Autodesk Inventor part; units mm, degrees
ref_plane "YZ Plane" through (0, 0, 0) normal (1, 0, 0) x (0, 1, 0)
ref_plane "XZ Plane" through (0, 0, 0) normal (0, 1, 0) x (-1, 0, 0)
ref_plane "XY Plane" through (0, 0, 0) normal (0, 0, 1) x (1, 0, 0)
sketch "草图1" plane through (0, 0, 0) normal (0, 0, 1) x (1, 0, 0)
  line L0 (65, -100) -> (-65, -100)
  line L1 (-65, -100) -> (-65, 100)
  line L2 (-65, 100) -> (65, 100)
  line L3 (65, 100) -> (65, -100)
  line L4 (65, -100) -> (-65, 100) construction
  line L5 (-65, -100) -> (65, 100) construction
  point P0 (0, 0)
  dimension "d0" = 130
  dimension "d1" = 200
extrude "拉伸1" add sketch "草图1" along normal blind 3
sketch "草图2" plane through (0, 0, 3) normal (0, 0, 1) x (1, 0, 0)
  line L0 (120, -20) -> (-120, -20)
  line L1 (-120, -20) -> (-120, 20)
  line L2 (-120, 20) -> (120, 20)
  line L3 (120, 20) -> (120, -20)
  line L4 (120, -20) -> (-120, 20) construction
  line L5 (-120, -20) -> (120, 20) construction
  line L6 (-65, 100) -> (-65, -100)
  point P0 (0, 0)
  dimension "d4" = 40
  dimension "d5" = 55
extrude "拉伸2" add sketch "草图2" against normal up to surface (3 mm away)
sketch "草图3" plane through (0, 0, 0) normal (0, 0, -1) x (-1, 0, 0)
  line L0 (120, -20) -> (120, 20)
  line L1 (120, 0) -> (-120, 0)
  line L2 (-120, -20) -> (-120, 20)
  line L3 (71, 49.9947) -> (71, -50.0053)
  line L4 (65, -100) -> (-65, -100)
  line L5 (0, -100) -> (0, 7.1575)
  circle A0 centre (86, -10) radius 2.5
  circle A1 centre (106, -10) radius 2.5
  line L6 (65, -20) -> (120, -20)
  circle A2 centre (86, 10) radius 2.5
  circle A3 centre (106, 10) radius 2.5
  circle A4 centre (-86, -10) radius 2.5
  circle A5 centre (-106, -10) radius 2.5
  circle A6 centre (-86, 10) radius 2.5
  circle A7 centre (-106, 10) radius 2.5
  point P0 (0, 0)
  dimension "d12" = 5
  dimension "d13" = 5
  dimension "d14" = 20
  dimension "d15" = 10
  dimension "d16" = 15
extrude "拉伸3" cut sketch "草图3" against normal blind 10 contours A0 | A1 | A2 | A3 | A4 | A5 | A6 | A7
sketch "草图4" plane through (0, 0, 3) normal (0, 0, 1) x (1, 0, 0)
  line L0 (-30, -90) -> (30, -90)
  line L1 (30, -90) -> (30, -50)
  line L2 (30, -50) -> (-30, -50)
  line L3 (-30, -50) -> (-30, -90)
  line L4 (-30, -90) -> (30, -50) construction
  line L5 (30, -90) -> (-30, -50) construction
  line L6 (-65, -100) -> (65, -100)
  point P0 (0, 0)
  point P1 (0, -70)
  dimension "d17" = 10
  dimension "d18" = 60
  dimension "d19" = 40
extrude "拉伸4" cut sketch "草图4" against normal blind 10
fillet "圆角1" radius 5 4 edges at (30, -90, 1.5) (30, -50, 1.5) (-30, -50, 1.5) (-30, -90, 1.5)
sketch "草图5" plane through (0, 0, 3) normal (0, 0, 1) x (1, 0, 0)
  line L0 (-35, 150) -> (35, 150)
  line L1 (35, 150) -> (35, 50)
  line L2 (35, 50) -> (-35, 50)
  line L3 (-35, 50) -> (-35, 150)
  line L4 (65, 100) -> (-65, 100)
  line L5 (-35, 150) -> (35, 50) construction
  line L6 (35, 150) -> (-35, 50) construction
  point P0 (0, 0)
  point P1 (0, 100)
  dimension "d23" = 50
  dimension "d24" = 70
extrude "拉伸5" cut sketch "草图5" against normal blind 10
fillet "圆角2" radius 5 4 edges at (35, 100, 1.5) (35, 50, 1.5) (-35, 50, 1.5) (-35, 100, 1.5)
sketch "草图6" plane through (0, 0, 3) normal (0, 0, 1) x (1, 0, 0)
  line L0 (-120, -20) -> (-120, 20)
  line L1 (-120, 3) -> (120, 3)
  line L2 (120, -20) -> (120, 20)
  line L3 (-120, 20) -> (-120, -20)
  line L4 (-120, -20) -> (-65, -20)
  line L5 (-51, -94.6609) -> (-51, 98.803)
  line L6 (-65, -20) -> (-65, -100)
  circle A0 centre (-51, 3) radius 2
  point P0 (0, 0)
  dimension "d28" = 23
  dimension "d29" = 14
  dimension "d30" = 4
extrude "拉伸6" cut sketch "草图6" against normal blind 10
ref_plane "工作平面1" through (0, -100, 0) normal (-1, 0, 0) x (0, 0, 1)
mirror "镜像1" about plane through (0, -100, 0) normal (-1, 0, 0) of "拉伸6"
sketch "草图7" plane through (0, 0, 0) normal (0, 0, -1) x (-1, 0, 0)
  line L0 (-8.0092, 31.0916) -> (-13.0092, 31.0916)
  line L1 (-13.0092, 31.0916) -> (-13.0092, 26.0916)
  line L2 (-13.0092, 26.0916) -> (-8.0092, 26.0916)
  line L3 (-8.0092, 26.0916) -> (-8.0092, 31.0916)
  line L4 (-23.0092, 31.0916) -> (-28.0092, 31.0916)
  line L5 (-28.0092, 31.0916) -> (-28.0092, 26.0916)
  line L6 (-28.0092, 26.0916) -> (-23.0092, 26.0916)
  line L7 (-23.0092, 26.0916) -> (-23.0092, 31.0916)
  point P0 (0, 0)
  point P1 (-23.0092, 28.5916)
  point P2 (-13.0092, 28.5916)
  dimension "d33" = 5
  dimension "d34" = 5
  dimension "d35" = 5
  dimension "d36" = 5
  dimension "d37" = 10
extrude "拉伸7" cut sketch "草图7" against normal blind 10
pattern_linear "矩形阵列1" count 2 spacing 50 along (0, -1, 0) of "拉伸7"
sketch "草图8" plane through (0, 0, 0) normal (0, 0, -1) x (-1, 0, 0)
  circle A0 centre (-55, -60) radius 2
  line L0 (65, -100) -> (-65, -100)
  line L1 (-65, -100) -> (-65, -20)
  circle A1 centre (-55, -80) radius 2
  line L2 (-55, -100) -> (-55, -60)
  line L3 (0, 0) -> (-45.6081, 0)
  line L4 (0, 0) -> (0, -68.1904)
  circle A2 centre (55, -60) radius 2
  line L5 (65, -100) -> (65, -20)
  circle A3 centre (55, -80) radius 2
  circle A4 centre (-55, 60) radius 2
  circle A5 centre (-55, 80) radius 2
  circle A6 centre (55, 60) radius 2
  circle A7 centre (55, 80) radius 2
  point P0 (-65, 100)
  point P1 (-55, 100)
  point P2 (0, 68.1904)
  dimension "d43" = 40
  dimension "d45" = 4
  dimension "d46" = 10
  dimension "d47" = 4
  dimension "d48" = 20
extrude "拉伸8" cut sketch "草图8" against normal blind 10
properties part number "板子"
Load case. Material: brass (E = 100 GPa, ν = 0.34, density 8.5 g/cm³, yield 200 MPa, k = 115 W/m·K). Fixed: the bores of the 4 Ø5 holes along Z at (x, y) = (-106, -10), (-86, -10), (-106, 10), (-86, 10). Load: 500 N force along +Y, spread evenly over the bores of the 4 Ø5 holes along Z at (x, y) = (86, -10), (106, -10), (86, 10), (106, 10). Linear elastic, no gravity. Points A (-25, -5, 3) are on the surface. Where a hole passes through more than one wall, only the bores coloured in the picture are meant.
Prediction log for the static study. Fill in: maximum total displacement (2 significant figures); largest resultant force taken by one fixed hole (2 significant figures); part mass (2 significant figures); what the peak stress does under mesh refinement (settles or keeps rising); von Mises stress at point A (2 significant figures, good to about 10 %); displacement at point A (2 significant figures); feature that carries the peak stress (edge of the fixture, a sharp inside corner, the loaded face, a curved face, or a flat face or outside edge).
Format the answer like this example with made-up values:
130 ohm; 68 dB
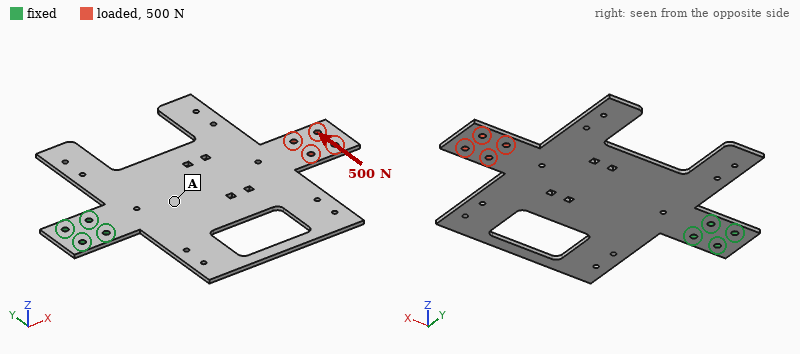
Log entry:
0.45 mm; 3.1 kN; 620 g; keeps rising; 12 MPa; 0.10 mm; edge of the fixture
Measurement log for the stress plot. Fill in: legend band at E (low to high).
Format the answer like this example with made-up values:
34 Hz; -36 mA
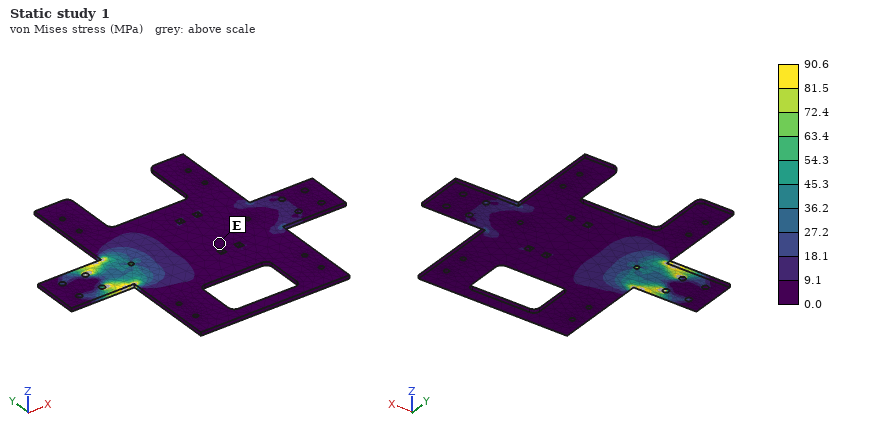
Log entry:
0.0 to 9.1 MPa
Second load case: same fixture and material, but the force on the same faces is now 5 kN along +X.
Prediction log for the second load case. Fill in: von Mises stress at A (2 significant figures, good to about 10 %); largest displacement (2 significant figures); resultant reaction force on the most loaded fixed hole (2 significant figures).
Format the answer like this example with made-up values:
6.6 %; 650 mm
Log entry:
27 MPa; 60 µm; 2.2 kN
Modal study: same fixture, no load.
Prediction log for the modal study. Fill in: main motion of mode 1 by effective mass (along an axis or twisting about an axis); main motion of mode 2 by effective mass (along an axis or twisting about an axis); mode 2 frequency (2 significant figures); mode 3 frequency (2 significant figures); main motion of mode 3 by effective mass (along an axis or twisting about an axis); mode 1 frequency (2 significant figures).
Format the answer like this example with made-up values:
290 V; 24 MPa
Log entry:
along Z; twisting about X; 79 Hz; 190 Hz; along Z; 36 Hz
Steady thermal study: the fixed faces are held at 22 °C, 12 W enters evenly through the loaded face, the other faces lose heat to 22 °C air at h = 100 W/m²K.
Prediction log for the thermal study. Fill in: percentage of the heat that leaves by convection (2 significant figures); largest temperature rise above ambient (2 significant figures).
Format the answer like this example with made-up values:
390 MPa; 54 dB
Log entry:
99 %; 20 K
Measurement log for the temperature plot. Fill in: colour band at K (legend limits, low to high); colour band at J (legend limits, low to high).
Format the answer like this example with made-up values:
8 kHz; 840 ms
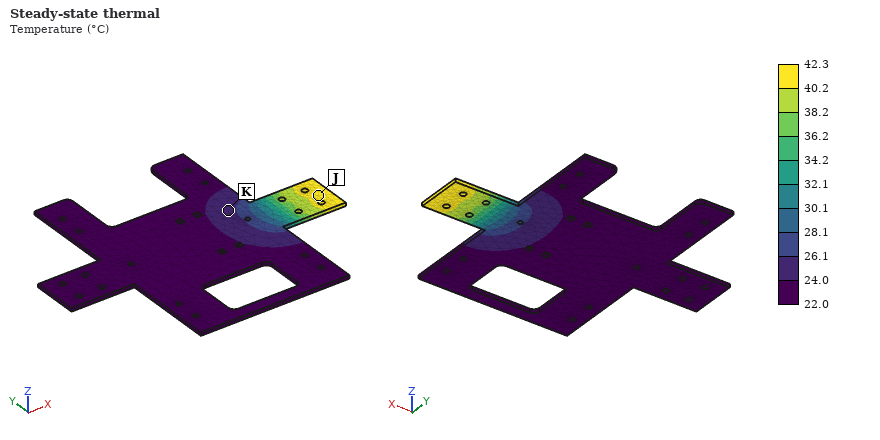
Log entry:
24.0 to 26.1 °C; 40.2 to 42.3 °C
